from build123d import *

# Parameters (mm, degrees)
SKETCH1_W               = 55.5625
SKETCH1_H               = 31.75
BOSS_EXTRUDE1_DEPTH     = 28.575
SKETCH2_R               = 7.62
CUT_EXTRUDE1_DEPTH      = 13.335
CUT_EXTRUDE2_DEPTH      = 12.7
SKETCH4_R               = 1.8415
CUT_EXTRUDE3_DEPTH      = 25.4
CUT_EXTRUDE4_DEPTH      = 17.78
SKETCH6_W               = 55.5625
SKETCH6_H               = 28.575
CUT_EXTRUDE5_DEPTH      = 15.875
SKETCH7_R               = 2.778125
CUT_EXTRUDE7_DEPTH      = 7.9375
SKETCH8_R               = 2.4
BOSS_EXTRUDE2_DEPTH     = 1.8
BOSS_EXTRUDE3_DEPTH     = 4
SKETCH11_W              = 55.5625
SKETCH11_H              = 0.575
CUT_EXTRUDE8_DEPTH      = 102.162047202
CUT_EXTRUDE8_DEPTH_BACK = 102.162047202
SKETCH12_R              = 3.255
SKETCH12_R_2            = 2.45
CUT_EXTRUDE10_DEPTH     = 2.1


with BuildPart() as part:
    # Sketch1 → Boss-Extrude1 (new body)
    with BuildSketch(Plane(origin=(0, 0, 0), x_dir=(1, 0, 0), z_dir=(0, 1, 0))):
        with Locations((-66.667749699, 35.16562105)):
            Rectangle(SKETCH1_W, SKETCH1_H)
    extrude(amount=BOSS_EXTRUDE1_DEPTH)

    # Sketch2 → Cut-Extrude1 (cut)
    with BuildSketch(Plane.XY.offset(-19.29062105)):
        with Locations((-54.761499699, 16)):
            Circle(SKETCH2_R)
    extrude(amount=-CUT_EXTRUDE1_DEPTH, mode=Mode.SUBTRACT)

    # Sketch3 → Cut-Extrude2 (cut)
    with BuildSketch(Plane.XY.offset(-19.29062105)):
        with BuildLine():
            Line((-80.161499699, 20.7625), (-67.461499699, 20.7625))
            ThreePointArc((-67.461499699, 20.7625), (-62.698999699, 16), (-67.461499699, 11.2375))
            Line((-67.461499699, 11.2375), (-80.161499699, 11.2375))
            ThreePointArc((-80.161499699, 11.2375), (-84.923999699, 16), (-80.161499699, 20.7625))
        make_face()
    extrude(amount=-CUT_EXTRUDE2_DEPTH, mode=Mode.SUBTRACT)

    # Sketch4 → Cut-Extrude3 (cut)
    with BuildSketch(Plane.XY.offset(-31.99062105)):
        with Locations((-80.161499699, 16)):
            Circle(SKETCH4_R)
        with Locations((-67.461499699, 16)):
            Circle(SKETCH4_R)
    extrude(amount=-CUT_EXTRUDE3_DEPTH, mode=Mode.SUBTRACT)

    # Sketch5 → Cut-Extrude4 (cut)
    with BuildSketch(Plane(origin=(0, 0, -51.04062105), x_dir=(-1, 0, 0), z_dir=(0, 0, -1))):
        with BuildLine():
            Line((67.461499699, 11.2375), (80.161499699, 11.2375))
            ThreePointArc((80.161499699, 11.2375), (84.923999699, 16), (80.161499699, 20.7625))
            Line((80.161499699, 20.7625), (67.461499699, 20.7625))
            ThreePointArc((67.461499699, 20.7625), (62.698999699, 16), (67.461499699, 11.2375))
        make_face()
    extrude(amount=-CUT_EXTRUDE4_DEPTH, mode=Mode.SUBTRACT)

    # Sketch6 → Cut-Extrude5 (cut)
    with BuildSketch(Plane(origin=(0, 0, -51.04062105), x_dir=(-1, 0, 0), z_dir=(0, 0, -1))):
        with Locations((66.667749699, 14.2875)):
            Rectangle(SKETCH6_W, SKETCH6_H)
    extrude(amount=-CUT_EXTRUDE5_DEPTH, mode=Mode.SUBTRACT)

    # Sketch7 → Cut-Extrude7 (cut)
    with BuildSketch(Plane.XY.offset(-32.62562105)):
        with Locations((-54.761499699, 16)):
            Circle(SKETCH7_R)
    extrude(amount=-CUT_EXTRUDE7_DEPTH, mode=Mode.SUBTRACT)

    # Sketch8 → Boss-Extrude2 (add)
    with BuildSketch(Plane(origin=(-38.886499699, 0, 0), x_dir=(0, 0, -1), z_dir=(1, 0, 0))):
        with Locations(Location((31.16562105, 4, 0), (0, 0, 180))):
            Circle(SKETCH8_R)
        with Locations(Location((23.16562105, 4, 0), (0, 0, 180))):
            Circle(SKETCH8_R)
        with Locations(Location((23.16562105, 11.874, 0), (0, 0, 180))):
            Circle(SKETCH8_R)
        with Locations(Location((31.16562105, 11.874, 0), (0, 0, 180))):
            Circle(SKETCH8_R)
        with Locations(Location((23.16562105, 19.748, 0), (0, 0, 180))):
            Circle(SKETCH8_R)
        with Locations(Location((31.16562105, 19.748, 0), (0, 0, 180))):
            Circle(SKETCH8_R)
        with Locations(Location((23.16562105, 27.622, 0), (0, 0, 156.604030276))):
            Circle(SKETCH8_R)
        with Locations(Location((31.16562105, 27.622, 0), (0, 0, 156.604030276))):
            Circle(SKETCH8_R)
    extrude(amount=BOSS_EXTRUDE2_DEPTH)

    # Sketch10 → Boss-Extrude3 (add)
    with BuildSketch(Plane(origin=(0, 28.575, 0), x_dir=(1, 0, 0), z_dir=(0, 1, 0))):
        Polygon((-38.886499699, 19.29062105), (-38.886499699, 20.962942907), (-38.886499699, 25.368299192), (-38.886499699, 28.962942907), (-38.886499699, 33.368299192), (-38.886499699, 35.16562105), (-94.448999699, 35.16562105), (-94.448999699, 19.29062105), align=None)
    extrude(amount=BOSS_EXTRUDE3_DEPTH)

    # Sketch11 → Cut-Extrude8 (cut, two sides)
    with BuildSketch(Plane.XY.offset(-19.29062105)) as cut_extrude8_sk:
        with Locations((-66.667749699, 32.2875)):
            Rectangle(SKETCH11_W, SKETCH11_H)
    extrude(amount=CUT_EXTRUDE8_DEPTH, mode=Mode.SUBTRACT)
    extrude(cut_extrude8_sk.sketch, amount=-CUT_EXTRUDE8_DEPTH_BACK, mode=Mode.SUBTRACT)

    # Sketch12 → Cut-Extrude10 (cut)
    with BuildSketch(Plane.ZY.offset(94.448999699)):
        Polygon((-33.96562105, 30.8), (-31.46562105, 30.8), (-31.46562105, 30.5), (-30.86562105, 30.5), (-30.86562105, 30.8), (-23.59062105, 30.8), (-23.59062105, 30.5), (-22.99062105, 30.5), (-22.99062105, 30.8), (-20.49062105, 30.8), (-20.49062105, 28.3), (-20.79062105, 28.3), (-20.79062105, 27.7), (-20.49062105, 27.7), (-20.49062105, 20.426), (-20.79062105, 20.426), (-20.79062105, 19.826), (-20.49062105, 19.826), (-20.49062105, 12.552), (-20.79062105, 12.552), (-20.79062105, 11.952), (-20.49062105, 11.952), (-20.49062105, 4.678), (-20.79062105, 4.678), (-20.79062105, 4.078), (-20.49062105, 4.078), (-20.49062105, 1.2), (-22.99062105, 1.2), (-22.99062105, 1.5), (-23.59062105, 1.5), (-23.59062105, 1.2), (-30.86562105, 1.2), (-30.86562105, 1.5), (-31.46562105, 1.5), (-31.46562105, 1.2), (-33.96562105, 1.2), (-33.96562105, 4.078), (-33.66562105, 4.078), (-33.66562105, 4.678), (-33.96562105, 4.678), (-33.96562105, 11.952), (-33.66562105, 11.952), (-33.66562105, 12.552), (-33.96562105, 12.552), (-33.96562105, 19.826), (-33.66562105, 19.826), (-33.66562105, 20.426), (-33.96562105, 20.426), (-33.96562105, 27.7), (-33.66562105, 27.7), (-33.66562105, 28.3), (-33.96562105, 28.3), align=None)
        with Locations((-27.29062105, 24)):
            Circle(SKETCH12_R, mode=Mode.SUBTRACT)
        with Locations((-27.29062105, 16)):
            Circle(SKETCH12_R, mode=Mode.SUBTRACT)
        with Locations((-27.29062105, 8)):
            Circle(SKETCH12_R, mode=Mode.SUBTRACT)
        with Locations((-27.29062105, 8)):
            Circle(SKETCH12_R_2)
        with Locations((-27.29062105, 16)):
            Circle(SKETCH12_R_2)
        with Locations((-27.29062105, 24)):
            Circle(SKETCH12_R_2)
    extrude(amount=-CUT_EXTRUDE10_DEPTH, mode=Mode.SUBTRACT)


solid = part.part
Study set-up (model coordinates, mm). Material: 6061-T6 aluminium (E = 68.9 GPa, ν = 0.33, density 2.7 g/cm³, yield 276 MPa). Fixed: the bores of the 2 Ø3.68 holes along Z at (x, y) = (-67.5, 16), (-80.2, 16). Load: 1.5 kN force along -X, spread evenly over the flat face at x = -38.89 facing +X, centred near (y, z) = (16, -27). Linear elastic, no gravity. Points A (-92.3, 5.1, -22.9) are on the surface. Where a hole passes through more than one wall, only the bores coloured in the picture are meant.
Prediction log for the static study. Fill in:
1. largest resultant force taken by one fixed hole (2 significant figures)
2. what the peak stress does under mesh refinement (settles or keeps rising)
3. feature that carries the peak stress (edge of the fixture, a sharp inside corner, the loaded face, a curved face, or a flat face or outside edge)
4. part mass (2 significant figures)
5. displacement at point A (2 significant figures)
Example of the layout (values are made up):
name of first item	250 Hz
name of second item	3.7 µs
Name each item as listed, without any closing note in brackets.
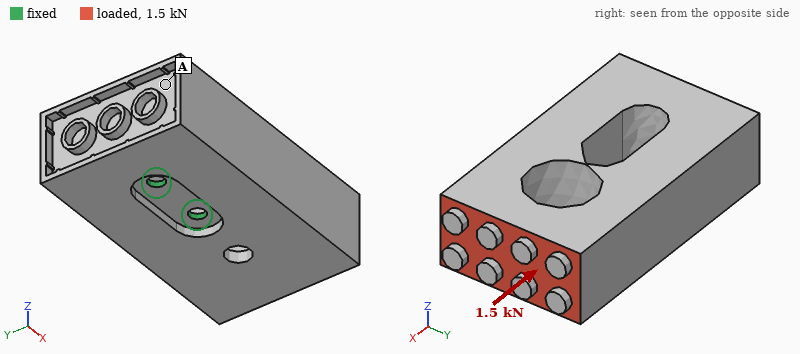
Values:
largest resultant force taken by one fixed hole	930 N
what the peak stress does under mesh refinement	keeps rising
feature that carries the peak stress	edge of the fixture
part mass	61 g
displacement at point A	33 µm
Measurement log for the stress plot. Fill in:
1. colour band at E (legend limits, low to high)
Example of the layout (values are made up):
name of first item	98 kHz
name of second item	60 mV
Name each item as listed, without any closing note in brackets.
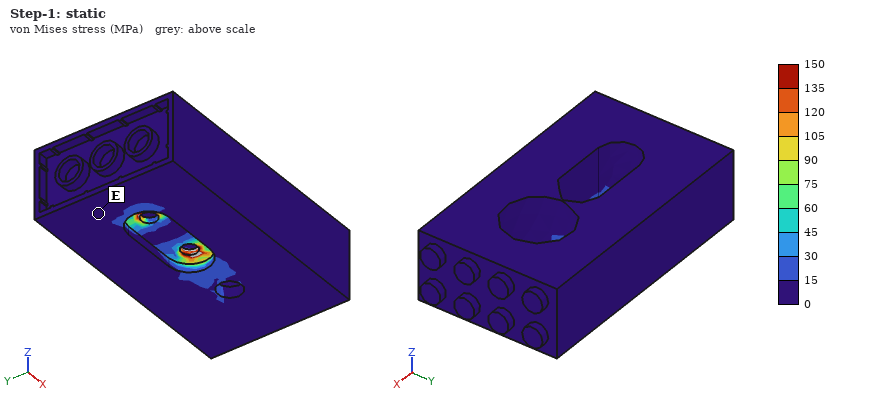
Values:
colour band at E	0 to 15 MPa
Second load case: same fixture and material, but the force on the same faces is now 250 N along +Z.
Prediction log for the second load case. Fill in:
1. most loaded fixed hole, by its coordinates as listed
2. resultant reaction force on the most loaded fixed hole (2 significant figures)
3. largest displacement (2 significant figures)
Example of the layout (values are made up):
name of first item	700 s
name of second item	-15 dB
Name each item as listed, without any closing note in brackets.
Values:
most loaded fixed hole, by its coordinates as listed	(-67.5, 16)
resultant reaction force on the most loaded fixed hole	680 N
largest displacement	72 µm
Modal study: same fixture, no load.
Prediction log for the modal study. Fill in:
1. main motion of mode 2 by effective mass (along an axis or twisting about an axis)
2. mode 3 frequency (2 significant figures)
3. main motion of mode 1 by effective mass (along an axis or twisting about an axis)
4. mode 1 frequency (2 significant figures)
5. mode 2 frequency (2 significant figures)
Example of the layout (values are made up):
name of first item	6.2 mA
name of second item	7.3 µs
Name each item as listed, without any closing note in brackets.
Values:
main motion of mode 2 by effective mass	along Z
mode 3 frequency	4500 Hz
main motion of mode 1 by effective mass	along Y
mode 1 frequency	1400 Hz
mode 2 frequency	2300 Hz
